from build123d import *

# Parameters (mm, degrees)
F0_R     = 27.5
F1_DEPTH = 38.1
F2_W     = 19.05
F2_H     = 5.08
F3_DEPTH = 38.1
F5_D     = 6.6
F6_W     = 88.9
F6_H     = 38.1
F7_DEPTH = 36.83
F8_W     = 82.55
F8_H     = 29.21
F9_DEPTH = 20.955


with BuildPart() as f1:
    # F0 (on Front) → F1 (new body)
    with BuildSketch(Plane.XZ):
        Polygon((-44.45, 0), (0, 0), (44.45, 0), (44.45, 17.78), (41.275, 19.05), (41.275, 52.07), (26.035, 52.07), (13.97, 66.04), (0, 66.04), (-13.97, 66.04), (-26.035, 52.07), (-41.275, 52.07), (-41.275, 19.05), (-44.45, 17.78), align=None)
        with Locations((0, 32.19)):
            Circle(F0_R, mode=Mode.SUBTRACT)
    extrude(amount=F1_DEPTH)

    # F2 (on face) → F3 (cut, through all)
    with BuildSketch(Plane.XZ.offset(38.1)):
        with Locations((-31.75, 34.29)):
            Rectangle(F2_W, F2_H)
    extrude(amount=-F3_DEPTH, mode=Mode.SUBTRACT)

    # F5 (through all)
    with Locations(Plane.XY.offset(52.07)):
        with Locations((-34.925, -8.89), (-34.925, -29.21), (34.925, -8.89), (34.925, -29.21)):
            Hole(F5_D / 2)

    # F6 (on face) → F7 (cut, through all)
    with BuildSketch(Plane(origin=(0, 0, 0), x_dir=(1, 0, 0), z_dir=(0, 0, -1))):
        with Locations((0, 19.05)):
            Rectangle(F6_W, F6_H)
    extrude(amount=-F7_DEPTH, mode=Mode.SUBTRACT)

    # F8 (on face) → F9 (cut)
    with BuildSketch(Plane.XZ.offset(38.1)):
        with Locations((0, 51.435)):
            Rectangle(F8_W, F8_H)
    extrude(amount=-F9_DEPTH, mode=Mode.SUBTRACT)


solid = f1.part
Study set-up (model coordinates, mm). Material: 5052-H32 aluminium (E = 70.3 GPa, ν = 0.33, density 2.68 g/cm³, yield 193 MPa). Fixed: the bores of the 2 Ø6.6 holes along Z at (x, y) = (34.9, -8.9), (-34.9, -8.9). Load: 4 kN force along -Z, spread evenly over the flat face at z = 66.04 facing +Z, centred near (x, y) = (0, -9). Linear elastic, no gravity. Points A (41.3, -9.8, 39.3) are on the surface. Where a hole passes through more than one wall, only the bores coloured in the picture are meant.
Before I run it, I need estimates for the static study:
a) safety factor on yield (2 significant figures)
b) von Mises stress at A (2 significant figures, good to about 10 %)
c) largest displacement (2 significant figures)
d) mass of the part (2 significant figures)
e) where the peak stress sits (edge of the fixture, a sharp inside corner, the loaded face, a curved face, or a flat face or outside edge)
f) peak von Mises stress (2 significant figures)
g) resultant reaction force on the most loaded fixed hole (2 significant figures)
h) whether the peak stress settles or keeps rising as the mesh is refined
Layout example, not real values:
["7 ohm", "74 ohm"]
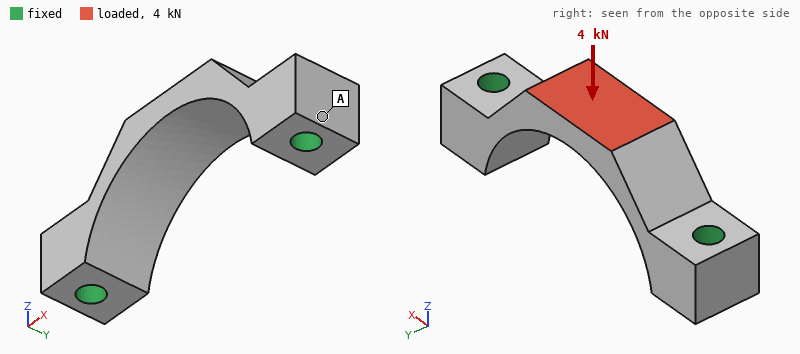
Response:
["3.1", "6.7 MPa", "33 µm", "38 g", "the loaded face", "63 MPa", "3.1 kN", "settles"]
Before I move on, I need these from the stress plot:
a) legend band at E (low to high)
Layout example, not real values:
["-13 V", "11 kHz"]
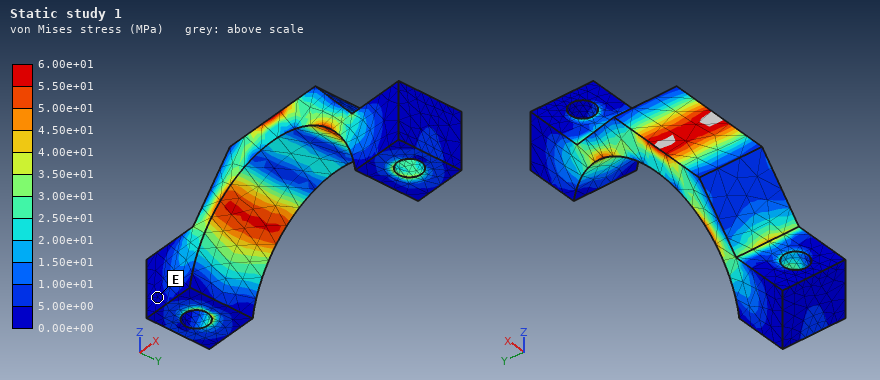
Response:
["0.00e+00 to 5.00e+00 MPa"]
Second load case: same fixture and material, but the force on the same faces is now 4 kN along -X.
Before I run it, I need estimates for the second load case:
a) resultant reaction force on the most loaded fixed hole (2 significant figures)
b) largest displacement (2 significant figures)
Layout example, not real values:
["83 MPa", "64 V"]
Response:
["2.3 kN", "21 µm"]
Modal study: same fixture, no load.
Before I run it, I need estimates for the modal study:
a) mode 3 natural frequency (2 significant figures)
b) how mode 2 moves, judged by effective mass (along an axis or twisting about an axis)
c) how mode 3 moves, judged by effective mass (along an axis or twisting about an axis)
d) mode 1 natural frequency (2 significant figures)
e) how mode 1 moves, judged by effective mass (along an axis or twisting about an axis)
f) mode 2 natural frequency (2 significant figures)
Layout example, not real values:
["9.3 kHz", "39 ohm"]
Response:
["19 kHz", "along X", "along Z", "8900 Hz", "along Y", "16 kHz"]
